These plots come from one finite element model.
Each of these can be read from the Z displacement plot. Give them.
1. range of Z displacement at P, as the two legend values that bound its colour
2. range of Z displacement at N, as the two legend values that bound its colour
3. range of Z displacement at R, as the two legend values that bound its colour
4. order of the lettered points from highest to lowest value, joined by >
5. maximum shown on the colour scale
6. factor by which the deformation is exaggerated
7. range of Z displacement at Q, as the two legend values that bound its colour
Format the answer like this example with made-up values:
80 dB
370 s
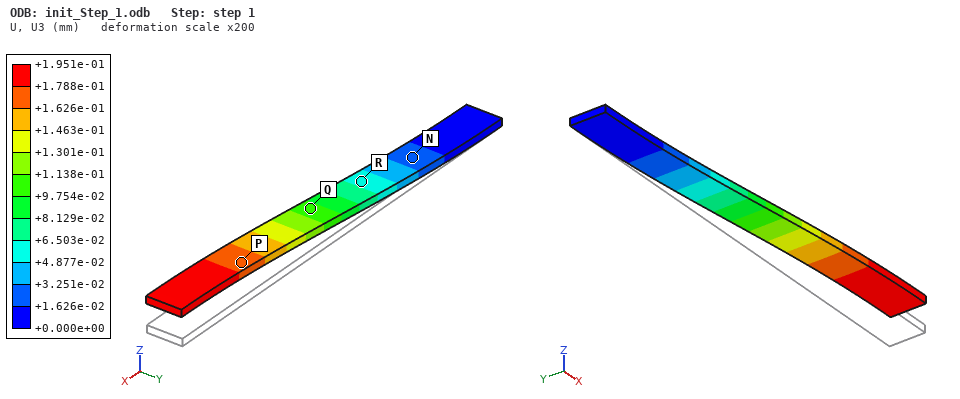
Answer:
+1.626e-01 to +1.788e-01 mm
+1.626e-02 to +3.251e-02 mm
+4.877e-02 to +6.503e-02 mm
P > Q > R > N
+1.951e-01 mm
200
+9.754e-02 to +1.138e-01 mm
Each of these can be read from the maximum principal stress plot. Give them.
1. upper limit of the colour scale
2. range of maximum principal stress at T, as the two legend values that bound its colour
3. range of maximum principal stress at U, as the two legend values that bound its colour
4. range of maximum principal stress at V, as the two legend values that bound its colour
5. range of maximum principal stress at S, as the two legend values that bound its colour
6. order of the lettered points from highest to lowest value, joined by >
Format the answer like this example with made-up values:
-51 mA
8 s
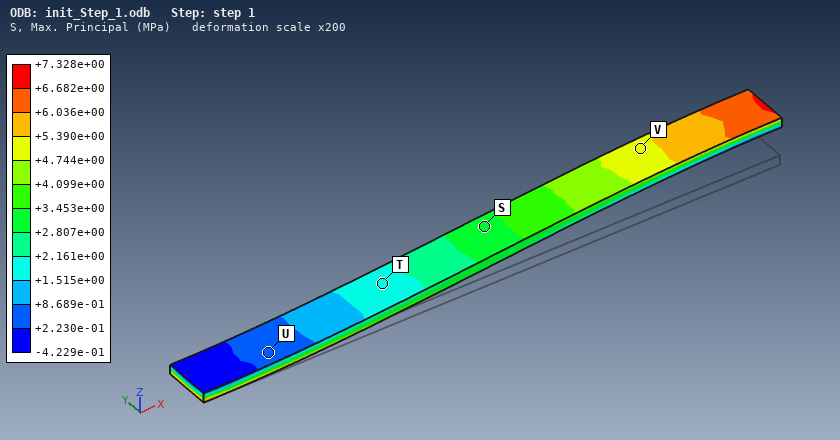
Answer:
+7.328e+00 MPa
+1.515e+00 to +2.161e+00 MPa
+2.230e-01 to +8.689e-01 MPa
+4.744e+00 to +5.390e+00 MPa
+2.807e+00 to +3.453e+00 MPa
V > S > T > U
